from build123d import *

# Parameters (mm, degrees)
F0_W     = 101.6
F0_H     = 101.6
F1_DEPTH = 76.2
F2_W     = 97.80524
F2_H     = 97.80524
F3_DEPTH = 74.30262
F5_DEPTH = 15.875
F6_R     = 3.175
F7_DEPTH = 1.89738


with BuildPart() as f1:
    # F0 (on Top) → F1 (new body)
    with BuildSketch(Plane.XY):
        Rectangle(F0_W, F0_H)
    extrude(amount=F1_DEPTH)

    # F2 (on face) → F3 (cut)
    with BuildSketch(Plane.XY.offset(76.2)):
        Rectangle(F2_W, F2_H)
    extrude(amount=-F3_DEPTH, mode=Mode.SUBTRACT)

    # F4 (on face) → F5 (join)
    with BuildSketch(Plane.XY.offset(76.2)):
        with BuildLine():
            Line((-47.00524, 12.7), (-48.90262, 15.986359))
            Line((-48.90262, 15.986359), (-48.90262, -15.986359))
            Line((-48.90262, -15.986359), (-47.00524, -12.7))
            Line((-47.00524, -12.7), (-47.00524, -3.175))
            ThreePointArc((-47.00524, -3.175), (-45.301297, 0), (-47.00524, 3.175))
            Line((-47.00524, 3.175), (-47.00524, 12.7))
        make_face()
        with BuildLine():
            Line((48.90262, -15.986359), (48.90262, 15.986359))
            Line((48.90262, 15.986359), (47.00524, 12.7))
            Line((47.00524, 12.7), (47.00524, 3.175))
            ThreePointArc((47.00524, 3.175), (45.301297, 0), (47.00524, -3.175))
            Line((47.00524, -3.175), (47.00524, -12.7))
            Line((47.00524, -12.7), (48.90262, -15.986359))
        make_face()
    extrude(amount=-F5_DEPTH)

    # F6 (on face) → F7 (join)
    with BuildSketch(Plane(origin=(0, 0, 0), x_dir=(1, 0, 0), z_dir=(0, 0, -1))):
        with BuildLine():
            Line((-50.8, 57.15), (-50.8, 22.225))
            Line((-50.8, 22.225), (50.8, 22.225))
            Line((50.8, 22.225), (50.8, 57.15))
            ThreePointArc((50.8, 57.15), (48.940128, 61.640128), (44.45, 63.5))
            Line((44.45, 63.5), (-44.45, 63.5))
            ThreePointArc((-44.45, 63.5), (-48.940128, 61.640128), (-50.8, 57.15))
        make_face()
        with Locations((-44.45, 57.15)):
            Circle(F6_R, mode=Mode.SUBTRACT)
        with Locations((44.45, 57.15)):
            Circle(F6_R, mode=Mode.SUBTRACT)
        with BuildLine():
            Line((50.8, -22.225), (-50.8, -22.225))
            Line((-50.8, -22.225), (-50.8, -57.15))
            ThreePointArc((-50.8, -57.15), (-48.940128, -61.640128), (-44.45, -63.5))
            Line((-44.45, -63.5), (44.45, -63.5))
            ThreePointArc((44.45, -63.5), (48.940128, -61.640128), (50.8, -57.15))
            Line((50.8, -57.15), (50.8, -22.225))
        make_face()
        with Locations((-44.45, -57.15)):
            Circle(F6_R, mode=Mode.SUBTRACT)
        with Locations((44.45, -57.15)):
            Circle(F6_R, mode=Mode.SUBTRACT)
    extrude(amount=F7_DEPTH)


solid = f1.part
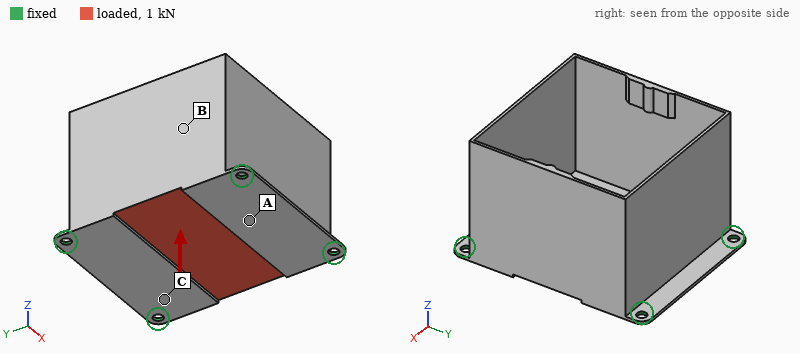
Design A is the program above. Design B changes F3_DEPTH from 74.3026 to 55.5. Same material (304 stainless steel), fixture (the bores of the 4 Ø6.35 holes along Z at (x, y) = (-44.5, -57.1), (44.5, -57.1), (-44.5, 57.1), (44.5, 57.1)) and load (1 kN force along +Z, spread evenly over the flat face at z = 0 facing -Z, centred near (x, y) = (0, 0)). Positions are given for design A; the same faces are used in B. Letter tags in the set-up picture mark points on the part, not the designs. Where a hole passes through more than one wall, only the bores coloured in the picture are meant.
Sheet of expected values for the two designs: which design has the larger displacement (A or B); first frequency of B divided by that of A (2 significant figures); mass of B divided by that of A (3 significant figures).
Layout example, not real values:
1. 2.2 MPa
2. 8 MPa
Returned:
1. A
2. 1.3
3. 2.93
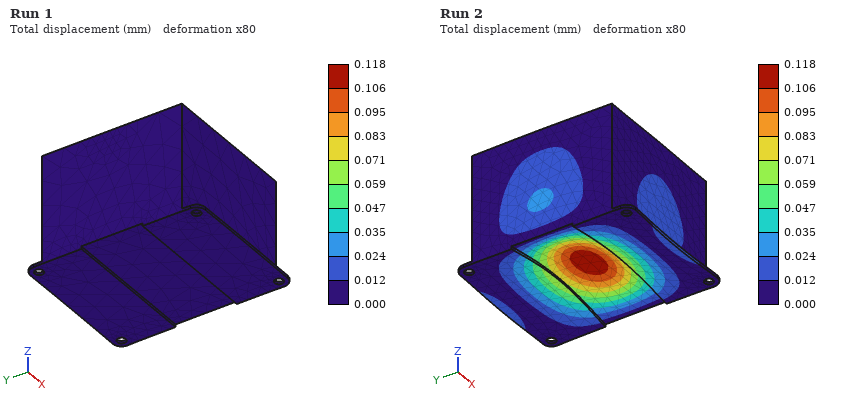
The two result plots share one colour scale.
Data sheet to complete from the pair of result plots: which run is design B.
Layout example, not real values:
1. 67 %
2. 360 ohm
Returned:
1. Run 1
